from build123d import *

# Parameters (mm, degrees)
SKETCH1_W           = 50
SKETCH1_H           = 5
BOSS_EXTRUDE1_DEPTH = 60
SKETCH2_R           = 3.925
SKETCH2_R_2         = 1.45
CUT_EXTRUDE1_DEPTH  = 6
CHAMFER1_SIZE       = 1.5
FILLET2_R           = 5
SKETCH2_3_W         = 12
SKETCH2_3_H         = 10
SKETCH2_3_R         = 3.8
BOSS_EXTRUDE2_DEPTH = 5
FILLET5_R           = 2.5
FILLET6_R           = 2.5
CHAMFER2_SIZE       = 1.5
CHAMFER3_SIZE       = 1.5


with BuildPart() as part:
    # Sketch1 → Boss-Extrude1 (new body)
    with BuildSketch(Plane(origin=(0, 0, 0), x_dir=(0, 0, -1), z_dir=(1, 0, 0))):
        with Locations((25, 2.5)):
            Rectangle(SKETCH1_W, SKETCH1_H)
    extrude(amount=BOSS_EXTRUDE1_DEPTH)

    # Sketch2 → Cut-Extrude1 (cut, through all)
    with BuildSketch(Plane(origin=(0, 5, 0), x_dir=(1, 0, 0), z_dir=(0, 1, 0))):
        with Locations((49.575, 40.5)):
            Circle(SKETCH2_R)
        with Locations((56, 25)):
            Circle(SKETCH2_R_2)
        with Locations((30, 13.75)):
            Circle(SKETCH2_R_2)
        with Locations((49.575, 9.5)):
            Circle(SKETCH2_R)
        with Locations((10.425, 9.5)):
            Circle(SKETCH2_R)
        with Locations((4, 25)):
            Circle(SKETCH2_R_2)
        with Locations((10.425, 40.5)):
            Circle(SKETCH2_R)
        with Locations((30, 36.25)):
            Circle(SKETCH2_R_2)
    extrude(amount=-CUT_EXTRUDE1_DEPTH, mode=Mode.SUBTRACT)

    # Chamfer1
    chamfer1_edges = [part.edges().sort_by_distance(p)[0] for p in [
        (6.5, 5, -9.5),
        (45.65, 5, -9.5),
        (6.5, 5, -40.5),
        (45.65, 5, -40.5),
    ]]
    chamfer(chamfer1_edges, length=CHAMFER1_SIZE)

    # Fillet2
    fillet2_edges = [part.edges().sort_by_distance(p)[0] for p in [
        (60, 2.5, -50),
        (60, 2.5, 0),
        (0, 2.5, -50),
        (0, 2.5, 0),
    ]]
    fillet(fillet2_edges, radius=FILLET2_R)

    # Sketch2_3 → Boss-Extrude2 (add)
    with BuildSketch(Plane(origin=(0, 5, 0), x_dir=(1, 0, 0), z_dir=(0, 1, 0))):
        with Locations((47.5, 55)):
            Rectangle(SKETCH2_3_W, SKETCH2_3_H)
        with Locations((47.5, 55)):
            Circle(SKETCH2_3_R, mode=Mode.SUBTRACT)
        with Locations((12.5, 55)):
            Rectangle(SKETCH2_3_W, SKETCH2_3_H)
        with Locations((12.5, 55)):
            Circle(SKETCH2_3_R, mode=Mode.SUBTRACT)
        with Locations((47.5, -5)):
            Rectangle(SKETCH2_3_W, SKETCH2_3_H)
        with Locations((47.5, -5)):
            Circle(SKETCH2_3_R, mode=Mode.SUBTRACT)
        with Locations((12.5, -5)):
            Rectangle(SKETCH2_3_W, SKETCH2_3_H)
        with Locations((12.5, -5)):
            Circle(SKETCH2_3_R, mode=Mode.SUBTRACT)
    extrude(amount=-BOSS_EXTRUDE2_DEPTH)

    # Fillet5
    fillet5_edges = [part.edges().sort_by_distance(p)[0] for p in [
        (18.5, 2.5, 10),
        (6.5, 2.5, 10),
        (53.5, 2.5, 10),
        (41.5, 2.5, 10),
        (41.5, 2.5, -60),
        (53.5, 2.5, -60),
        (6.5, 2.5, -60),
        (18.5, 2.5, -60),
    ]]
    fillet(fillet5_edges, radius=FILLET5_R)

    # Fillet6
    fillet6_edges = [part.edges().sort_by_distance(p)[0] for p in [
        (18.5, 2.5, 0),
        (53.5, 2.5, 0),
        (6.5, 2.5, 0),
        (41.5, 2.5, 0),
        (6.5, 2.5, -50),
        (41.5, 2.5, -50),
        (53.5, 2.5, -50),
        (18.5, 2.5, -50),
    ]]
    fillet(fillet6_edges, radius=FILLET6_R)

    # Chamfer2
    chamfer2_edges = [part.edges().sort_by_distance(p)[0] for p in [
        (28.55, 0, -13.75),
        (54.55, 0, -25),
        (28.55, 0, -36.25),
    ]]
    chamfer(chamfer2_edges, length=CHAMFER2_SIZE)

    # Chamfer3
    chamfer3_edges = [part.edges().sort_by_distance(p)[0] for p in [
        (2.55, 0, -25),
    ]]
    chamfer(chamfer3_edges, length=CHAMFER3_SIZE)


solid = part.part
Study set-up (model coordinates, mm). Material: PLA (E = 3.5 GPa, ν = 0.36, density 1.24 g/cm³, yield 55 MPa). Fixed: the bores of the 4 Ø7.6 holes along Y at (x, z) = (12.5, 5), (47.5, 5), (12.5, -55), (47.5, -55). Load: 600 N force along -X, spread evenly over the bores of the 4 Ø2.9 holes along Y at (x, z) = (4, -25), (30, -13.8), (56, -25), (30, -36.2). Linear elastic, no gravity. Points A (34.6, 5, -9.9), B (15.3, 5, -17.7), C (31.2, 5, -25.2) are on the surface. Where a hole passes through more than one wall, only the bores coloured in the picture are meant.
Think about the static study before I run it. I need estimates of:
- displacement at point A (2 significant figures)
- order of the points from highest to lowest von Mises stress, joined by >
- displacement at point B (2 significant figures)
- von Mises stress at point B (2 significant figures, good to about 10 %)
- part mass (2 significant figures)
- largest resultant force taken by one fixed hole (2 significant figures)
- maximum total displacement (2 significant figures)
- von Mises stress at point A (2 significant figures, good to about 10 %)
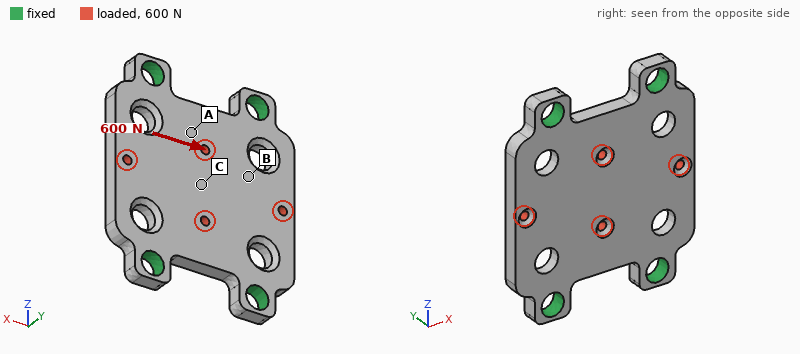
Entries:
23 µm
A > B > C
32 µm
1.6 MPa
19 g
160 N
55 µm
3.9 MPa
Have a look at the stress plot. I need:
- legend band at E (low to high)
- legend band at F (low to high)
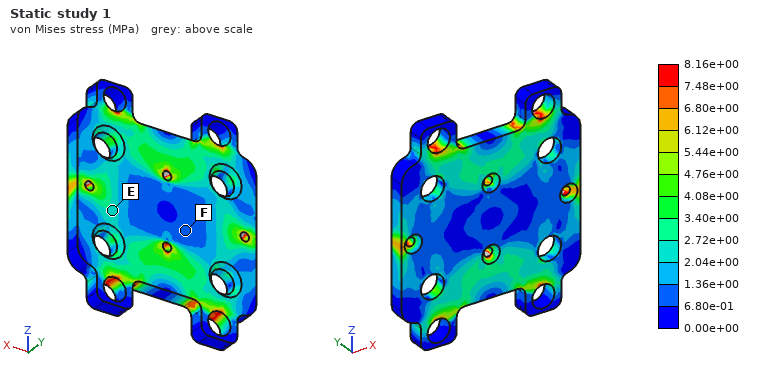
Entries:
2.04e+00 to 2.72e+00 MPa
6.80e-01 to 1.36e+00 MPa
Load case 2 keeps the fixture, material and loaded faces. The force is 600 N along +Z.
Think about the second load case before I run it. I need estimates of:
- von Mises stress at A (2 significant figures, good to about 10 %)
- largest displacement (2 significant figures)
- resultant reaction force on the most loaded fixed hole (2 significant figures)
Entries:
2.0 MPa
21 µm
150 N
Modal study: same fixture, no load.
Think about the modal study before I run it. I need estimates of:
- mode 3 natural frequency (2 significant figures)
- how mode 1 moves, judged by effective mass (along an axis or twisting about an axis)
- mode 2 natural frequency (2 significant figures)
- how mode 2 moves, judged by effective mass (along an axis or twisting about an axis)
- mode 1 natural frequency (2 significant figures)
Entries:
3700 Hz
along Y
2600 Hz
twisting about Z
2200 Hz
